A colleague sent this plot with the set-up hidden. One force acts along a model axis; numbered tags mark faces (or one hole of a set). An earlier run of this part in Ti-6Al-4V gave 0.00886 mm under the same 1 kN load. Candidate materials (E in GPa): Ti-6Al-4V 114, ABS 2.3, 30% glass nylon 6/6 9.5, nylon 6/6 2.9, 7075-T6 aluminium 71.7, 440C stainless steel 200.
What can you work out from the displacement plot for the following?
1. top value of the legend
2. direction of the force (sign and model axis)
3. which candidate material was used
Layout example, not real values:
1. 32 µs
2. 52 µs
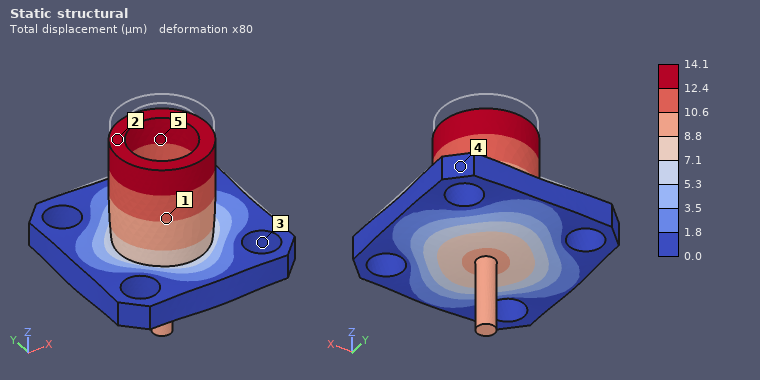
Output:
1. 14.1 µm
2. -Z
3. 7075-T6 aluminium
